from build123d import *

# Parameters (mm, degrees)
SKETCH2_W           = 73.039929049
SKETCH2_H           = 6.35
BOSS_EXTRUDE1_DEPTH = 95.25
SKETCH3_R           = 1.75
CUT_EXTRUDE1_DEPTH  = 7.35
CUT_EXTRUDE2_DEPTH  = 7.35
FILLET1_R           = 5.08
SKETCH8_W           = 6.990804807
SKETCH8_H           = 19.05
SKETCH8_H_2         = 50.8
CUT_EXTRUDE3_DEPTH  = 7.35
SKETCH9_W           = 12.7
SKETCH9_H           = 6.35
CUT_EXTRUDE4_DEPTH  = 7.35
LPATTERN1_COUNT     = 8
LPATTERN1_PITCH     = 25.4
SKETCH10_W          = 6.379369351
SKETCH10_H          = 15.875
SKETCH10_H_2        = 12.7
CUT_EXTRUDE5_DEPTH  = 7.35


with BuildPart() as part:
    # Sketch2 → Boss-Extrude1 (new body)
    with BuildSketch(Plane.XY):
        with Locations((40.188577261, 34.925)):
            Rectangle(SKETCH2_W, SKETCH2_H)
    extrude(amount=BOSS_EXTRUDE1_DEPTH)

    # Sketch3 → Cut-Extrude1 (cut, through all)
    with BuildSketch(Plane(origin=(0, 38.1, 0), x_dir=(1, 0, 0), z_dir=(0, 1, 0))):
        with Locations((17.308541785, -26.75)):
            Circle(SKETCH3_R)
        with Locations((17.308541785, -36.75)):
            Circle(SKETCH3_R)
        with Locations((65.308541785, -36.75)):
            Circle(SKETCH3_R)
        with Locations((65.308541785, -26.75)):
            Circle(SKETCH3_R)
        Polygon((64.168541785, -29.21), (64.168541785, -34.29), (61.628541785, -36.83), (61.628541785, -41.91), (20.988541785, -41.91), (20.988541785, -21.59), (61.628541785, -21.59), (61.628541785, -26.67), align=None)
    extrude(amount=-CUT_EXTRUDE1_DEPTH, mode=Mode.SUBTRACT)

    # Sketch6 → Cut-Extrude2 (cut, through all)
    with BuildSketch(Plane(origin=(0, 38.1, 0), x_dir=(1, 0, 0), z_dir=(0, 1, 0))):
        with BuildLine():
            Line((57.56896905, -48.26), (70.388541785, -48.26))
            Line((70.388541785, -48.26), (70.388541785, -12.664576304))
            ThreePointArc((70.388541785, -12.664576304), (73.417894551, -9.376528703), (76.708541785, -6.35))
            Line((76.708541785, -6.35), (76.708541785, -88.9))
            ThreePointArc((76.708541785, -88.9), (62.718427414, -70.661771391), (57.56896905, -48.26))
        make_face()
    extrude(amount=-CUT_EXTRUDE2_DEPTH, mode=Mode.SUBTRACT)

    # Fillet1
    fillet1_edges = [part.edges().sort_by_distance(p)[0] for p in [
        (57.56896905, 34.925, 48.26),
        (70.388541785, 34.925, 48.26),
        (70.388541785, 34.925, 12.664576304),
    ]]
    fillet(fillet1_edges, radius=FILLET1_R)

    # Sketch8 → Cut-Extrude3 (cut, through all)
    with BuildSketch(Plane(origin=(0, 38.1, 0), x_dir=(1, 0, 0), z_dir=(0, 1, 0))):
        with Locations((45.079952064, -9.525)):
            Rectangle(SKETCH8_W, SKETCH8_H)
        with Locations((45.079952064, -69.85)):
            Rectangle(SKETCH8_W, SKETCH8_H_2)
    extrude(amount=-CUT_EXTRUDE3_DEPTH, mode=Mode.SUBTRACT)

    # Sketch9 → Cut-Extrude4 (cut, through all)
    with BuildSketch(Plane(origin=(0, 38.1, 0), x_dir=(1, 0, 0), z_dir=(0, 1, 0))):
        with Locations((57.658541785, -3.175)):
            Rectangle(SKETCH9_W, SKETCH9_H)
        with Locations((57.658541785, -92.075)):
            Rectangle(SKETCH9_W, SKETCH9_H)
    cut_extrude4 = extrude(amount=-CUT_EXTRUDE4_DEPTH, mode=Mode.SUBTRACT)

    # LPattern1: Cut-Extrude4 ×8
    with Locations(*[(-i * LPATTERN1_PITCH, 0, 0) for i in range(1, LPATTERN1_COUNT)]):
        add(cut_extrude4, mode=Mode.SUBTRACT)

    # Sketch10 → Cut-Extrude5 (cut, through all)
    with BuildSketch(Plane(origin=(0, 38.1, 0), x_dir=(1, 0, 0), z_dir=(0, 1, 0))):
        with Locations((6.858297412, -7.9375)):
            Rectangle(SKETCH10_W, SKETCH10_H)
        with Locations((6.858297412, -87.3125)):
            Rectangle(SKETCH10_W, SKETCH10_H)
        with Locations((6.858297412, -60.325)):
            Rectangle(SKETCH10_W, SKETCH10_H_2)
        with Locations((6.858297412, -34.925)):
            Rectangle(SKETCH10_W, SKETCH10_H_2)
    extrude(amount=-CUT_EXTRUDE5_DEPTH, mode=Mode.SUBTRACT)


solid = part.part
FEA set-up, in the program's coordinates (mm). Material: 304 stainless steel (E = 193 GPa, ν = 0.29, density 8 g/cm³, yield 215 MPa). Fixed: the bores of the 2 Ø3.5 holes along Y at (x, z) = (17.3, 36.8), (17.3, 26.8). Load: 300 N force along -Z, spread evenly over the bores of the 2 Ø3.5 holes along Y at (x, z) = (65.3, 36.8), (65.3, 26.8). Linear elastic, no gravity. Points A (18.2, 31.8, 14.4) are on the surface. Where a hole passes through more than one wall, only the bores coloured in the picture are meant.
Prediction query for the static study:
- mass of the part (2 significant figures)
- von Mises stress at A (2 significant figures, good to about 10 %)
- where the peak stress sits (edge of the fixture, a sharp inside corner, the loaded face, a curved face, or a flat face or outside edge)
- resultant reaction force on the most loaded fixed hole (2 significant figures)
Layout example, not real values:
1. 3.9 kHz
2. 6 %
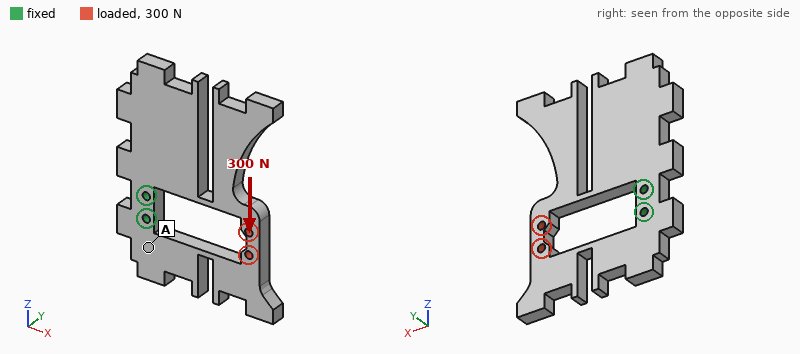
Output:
1. 210 g
2. 12 MPa
3. the loaded face
4. 860 N
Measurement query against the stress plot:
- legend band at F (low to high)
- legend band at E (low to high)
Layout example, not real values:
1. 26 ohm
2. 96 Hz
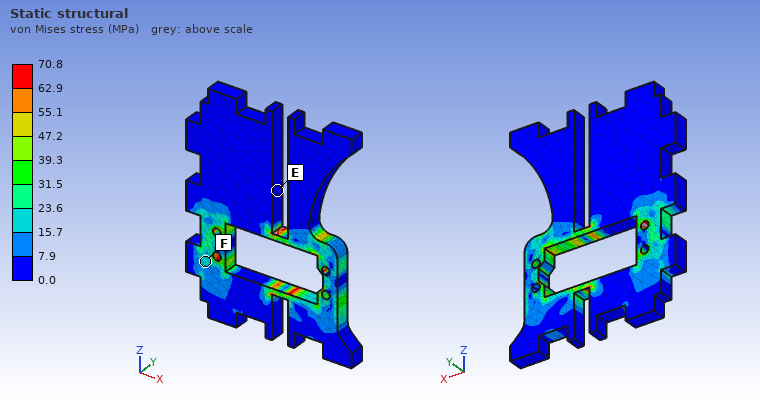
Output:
1. 15.7 to 23.6 MPa
2. 0.0 to 7.9 MPa
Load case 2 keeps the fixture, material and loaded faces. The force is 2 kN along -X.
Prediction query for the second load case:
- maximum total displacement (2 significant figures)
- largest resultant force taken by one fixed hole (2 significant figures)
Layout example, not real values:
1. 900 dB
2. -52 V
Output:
1. 32 µm
2. 1.3 kN
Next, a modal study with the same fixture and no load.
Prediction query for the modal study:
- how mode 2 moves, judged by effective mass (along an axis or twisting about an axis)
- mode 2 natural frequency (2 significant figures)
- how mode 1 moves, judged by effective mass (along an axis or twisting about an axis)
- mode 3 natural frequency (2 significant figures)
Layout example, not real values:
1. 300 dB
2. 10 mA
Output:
1. along Y
2. 910 Hz
3. along Y
4. 1000 Hz
